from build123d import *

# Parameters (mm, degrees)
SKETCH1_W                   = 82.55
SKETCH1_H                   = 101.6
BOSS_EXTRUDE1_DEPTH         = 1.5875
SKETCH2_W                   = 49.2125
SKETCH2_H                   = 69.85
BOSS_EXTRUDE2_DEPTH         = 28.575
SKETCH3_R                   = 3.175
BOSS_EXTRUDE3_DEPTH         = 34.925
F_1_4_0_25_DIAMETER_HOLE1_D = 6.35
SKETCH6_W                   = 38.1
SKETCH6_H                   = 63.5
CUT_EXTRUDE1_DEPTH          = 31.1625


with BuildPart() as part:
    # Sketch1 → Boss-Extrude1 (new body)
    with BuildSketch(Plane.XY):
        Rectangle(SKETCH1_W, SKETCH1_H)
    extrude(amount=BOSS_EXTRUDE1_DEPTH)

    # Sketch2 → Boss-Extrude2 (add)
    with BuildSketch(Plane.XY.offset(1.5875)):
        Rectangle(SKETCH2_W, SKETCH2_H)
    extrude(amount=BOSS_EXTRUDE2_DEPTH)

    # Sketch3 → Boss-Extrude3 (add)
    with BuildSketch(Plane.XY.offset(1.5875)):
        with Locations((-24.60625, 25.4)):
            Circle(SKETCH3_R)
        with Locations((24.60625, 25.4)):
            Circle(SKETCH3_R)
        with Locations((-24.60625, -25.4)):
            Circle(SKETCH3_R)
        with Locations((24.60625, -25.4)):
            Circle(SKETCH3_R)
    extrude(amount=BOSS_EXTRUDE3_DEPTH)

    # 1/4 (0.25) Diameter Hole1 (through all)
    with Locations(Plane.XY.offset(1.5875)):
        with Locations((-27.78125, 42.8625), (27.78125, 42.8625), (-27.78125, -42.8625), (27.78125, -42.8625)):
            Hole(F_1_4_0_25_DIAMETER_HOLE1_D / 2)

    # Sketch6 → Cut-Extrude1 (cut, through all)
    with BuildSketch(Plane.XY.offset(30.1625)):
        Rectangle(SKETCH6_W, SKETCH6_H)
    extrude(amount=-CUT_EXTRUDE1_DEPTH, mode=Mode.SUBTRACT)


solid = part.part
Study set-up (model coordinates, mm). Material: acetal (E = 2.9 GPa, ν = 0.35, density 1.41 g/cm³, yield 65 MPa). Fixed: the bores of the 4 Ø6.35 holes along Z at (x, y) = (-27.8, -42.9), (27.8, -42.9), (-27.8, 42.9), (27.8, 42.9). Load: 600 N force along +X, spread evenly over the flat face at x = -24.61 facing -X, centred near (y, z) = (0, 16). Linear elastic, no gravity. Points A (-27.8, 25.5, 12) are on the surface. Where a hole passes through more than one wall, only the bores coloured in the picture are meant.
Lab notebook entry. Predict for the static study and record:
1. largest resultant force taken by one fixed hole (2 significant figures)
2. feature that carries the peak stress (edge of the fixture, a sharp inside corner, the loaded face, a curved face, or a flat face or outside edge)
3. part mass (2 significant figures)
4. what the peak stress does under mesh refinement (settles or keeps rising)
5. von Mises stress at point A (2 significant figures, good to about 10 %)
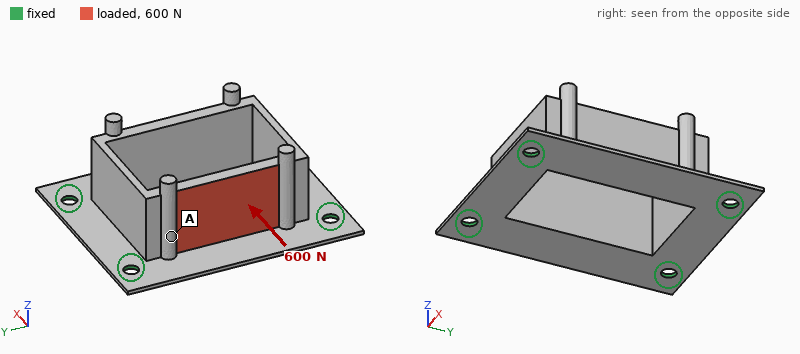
190 N
edge of the fixture
58 g
keeps rising
7.2 MPa
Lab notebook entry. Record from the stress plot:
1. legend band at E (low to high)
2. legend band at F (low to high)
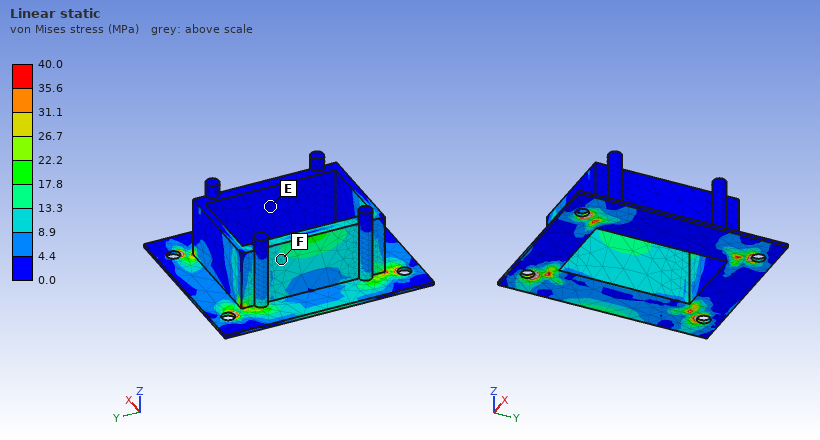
0.0 to 4.4 MPa
8.9 to 13.3 MPa
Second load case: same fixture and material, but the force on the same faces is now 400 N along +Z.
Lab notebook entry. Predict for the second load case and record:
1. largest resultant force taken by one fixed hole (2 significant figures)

240 N
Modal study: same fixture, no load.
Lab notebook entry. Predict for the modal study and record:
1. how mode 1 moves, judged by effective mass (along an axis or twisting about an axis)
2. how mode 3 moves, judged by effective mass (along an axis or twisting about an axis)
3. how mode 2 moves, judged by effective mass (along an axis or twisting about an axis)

along X
along Y
along Z
